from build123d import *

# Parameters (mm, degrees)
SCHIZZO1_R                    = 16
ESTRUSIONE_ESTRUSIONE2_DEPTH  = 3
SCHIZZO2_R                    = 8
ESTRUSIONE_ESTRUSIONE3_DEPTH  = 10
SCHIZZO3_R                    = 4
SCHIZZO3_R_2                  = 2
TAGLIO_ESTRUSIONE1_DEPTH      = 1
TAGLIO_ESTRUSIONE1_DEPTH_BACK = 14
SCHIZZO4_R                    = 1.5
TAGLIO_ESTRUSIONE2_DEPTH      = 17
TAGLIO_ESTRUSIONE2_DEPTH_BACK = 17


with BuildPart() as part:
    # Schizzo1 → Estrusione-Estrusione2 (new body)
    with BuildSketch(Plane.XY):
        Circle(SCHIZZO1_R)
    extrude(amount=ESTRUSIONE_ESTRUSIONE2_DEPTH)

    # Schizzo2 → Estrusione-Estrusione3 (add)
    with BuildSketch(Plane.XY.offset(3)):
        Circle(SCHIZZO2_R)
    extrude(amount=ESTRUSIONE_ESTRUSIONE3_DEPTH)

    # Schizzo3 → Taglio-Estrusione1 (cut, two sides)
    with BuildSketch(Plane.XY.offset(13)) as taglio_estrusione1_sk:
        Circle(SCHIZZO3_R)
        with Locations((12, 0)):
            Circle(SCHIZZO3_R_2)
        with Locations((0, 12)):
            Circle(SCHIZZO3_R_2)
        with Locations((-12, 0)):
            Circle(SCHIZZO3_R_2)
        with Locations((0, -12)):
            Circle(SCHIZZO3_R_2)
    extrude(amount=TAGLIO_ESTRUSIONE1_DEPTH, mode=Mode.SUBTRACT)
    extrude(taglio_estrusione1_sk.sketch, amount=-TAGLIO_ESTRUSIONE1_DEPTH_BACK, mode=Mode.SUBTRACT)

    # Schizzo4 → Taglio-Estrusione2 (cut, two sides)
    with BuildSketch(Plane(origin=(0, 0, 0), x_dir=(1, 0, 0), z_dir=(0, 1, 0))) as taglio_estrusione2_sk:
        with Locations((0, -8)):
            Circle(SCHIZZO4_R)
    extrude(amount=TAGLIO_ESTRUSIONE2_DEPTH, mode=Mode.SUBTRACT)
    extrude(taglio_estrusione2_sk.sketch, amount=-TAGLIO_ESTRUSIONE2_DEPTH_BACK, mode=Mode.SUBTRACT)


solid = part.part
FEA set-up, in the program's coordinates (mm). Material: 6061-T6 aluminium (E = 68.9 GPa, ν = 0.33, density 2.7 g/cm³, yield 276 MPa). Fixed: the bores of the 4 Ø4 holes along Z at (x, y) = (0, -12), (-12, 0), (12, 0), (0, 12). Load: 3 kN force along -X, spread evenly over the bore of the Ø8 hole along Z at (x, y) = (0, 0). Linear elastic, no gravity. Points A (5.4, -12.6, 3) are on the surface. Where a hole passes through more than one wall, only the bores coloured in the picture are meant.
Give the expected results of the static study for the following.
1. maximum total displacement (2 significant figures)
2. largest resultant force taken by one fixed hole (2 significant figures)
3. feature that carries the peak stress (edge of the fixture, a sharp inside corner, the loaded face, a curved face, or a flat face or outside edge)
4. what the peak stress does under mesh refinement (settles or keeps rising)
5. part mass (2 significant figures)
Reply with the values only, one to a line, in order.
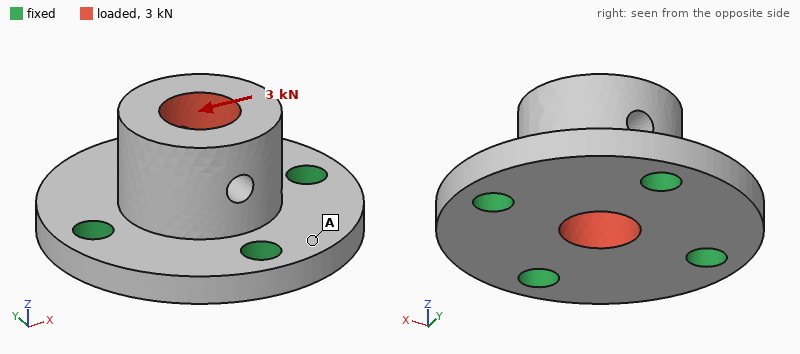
20 µm
1.2 kN
edge of the fixture
keeps rising
9.6 g
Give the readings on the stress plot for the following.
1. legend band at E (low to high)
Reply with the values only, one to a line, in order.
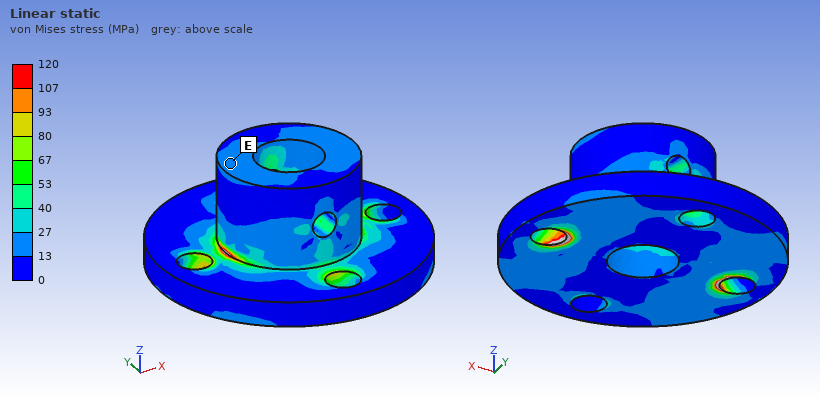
13 to 27 MPa
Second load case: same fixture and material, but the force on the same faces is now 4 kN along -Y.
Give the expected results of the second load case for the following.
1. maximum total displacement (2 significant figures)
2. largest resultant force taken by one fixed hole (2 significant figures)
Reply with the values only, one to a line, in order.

25 µm
1.6 kN
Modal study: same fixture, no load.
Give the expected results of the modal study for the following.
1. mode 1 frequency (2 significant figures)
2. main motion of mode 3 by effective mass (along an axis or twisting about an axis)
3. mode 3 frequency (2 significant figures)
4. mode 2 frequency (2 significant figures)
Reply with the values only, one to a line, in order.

31 kHz
along Z
38 kHz
31 kHz
